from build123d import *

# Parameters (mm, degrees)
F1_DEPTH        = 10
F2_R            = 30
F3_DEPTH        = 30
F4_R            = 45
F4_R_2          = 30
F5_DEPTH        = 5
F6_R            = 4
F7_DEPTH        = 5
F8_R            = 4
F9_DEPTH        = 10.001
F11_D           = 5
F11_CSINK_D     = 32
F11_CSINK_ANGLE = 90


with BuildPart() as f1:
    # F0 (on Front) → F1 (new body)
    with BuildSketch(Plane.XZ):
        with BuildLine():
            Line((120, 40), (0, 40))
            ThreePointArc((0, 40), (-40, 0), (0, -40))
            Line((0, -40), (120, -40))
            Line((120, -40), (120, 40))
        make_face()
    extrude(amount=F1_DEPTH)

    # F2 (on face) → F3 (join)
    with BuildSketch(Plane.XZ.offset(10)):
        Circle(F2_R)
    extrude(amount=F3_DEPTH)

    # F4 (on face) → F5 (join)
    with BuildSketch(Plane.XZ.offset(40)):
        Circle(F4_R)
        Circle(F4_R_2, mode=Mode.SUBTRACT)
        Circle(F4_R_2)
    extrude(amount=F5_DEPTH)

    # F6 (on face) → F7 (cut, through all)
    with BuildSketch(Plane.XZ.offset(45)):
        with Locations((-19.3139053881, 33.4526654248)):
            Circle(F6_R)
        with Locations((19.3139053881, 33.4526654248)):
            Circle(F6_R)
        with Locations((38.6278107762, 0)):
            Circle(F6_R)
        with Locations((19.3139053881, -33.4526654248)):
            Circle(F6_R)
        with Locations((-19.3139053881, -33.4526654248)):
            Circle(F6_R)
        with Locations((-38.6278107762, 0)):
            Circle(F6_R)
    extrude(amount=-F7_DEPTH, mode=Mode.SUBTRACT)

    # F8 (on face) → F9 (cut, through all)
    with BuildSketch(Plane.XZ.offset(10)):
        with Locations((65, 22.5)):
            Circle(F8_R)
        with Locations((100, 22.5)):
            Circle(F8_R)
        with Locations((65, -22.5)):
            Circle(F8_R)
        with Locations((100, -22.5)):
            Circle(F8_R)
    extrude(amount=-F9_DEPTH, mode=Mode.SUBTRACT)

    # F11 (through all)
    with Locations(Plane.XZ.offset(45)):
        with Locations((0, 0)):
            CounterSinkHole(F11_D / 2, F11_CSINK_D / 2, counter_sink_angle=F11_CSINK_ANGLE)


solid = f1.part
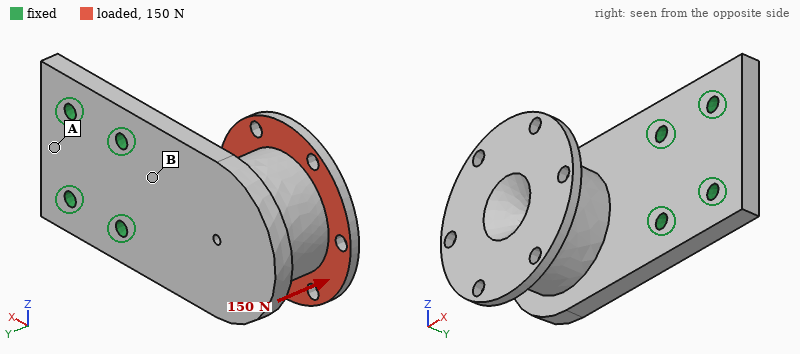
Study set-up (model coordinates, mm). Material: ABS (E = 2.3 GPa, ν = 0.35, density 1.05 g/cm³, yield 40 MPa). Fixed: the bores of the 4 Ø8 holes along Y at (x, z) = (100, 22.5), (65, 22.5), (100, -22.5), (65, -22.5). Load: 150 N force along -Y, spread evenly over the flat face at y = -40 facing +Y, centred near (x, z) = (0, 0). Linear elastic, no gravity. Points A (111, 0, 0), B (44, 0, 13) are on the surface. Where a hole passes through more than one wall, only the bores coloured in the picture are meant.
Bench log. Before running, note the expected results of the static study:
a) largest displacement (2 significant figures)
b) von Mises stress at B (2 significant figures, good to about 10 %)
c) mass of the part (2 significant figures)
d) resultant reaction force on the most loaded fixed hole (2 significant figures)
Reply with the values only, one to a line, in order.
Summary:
1.8 mm
4.3 MPa
240 g
110 N
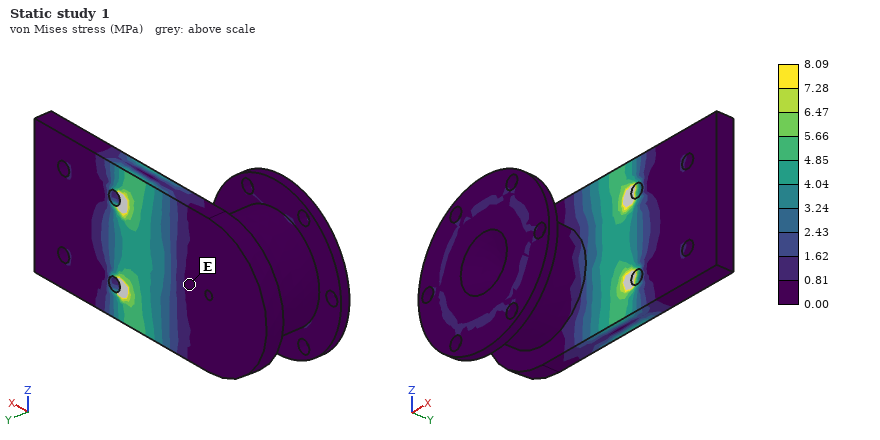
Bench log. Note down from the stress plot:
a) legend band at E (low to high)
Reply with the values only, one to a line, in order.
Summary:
0.00 to 0.81 MPa
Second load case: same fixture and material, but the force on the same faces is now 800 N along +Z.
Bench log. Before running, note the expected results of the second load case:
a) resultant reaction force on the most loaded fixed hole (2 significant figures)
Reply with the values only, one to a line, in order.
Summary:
1.1 kN
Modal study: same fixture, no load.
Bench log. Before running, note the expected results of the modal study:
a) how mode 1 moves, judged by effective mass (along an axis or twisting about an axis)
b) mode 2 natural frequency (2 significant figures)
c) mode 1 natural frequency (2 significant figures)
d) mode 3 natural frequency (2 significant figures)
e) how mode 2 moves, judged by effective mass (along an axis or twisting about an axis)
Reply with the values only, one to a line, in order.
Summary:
along Y
420 Hz
140 Hz
920 Hz
along Z
